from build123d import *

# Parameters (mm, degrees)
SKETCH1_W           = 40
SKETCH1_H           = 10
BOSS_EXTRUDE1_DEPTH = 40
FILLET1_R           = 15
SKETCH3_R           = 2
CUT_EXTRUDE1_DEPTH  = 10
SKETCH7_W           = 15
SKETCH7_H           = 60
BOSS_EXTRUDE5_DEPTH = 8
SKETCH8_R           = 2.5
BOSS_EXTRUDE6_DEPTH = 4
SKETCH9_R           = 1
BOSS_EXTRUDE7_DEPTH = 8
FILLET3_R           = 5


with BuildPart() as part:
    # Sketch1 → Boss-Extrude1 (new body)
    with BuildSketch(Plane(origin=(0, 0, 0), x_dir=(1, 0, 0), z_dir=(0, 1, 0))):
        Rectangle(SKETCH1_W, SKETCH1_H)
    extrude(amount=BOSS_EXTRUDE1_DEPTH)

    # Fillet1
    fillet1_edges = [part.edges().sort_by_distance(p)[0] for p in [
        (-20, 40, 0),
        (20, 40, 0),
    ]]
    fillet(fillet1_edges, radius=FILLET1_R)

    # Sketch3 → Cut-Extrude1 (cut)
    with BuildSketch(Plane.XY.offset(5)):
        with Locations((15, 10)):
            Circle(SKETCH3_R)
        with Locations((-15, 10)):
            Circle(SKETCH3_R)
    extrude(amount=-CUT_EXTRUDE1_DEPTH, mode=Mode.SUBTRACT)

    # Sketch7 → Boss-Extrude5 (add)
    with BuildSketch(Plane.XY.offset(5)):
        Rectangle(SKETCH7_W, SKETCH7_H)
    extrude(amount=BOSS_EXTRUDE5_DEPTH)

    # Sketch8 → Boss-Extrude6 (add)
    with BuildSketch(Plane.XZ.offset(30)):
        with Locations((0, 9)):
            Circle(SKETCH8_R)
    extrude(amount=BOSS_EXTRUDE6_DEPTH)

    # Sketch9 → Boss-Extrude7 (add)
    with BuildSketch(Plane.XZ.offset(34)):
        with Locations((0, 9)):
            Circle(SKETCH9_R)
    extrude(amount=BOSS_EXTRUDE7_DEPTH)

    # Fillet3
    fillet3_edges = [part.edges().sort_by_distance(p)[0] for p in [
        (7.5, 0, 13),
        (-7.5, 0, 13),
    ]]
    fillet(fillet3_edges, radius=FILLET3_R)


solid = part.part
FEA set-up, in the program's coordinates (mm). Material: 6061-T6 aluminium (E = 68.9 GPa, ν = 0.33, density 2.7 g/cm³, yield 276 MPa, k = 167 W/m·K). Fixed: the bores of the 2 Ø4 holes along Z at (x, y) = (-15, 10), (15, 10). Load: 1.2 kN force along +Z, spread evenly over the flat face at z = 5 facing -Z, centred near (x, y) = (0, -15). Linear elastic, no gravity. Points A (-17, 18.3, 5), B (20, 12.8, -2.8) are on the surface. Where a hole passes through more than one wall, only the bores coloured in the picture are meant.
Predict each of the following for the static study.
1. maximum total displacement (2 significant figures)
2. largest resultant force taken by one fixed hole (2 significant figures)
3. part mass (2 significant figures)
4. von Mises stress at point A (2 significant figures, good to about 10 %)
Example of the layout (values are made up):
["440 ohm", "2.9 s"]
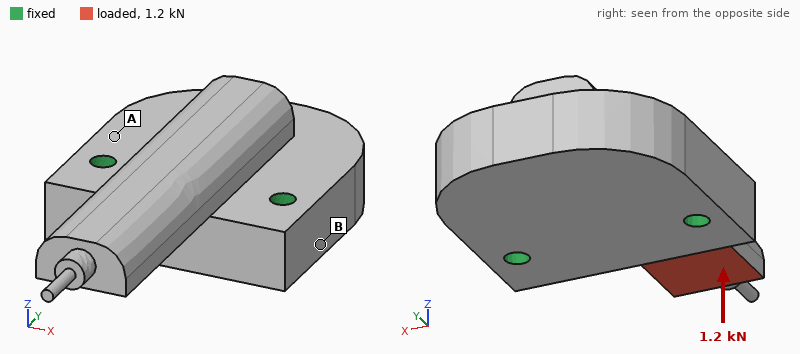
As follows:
["0.33 mm", "750 N", "58 g", "19 MPa"]
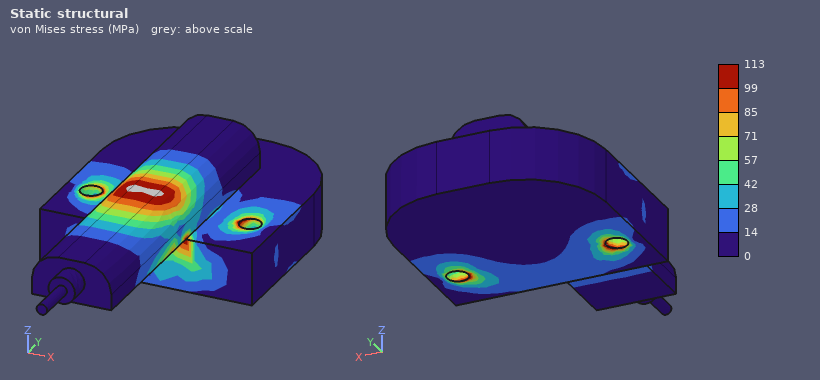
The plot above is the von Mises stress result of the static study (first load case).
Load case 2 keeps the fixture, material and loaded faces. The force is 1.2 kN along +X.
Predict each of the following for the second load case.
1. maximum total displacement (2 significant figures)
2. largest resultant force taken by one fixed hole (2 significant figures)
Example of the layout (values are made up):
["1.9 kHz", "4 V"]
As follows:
["0.12 mm", "1.2 kN"]
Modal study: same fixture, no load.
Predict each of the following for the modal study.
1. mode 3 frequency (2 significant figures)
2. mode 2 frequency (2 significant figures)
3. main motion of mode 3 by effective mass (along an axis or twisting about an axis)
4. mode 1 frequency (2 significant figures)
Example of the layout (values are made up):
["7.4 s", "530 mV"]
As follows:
["8700 Hz", "7300 Hz", "along Z", "4300 Hz"]
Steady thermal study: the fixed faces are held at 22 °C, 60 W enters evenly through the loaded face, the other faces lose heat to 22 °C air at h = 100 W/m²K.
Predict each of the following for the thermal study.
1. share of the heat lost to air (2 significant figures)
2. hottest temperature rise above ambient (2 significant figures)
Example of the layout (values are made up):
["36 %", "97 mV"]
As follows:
["14 %", "70 K"]
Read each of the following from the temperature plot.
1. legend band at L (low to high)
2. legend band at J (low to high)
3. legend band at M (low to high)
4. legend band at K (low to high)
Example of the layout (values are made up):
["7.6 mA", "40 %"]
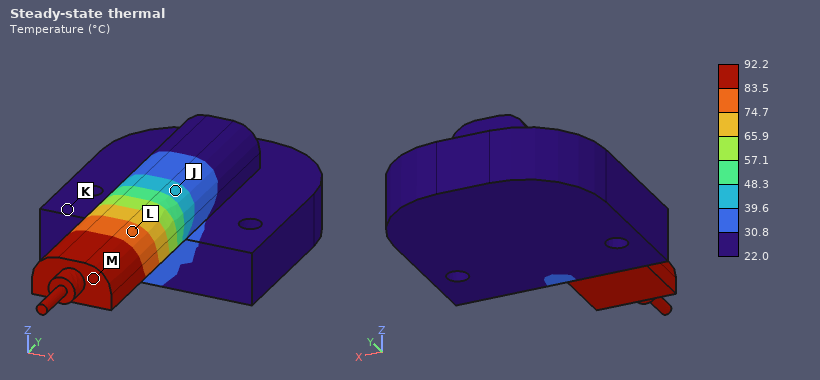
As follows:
["74.7 to 83.5 °C", "39.6 to 48.3 °C", "83.5 to 92.2 °C", "22.0 to 30.8 °C"]
